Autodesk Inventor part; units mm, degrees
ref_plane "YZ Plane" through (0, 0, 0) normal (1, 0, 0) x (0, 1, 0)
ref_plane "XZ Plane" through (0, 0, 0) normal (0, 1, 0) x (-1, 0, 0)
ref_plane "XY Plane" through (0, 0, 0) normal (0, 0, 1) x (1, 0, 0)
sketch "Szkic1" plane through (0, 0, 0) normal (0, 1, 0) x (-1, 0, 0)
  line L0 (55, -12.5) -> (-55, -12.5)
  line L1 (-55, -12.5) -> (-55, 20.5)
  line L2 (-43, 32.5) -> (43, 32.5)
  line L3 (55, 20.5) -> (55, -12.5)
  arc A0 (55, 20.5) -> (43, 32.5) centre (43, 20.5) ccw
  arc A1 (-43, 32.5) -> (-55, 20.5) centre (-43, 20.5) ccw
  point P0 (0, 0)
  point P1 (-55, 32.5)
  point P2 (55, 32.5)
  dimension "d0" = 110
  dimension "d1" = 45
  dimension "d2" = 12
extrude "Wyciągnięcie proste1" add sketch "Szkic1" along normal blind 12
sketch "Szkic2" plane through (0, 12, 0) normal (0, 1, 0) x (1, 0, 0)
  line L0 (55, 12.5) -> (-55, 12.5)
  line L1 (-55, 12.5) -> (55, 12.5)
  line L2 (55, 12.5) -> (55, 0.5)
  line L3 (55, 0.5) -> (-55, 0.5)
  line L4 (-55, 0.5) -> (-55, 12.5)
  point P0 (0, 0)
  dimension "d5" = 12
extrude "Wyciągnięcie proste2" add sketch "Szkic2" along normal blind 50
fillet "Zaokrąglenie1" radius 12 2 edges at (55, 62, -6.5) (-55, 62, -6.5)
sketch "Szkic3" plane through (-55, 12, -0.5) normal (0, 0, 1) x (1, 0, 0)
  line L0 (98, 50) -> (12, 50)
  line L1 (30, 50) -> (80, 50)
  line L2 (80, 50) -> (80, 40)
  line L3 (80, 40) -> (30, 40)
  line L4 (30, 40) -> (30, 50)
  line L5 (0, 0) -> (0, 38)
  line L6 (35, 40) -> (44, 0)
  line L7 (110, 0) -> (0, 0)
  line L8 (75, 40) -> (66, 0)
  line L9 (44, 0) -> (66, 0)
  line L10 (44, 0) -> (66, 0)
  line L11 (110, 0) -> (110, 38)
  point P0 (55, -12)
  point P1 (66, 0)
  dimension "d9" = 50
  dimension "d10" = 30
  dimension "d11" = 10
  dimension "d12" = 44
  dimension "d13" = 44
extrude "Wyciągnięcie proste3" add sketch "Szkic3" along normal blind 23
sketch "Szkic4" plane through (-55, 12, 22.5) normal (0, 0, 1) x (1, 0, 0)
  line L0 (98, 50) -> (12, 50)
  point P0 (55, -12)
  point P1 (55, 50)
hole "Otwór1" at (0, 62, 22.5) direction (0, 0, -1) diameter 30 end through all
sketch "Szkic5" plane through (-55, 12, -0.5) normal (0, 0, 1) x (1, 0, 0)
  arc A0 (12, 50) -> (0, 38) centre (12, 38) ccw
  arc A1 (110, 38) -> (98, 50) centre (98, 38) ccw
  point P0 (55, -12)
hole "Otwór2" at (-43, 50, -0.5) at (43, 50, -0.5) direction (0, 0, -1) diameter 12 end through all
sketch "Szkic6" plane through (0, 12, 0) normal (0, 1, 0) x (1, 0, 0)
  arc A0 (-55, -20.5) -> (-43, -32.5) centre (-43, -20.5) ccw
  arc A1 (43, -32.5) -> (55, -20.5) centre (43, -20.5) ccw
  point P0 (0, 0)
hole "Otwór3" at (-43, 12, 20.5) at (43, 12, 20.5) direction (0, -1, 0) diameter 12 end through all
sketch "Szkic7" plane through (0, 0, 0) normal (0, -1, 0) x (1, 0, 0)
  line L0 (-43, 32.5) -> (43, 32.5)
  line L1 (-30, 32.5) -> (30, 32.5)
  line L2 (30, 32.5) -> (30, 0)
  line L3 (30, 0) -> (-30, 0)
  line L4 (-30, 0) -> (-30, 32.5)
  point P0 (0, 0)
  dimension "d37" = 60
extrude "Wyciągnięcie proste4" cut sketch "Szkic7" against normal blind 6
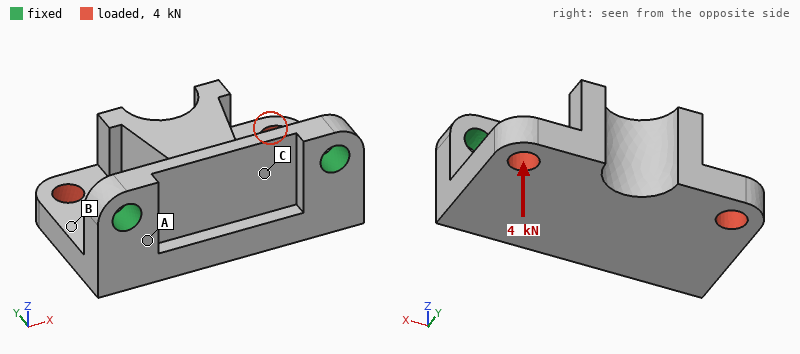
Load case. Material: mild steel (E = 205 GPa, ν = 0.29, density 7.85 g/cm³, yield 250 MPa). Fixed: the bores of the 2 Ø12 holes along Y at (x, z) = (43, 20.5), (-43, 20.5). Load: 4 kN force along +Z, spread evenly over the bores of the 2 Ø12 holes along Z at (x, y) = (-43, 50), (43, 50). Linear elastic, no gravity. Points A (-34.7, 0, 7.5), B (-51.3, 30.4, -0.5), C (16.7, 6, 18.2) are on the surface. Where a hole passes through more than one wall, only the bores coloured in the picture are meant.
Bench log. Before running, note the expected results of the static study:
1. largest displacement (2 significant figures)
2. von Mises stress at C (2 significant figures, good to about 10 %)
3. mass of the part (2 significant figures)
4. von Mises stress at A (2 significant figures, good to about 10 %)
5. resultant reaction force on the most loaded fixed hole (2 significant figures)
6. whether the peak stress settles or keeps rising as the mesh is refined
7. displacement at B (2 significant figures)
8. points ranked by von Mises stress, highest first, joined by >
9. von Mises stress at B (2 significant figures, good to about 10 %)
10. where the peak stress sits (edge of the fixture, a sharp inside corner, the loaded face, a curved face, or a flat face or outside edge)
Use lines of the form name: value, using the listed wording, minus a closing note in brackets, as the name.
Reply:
largest displacement: 0.13 mm
von Mises stress at C: 58 MPa
mass of the part: 1.1 kg
von Mises stress at A: 90 MPa
resultant reaction force on the most loaded fixed hole: 2.2 kN
whether the peak stress settles or keeps rising as the mesh is refined: keeps rising
displacement at B: 0.050 mm
points ranked by von Mises stress, highest first, joined by >: A > C > B
von Mises stress at B: 21 MPa
where the peak stress sits: edge of the fixture
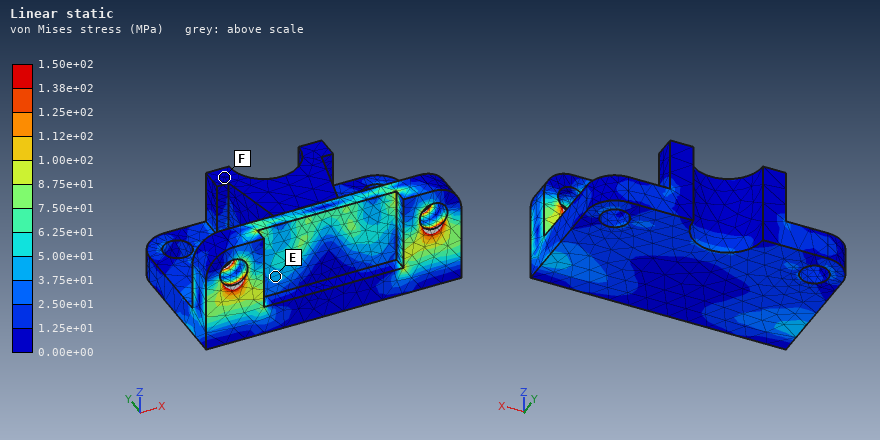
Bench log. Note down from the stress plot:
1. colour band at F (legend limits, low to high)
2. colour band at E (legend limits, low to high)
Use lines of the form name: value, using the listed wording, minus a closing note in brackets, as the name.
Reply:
colour band at F: 0.00e+00 to 1.25e+01 MPa
colour band at E: 3.75e+01 to 5.00e+01 MPa
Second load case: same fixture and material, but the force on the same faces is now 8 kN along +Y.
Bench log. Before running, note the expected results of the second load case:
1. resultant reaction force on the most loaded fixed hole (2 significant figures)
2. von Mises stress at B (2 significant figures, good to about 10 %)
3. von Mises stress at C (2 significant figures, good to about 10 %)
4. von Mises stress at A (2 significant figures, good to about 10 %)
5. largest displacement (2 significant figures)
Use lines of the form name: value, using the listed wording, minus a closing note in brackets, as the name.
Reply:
resultant reaction force on the most loaded fixed hole: 4.0 kN
von Mises stress at B: 19 MPa
von Mises stress at C: 27 MPa
von Mises stress at A: 66 MPa
largest displacement: 71 µm
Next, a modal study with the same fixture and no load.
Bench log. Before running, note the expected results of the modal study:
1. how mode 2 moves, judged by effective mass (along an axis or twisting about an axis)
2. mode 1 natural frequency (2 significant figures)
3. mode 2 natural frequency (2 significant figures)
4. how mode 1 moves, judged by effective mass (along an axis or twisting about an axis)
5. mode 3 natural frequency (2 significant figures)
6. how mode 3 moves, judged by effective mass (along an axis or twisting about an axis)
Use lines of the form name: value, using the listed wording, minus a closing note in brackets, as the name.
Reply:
how mode 2 moves, judged by effective mass: along X
mode 1 natural frequency: 1600 Hz
mode 2 natural frequency: 4100 Hz
how mode 1 moves, judged by effective mass: along Z
mode 3 natural frequency: 4400 Hz
how mode 3 moves, judged by effective mass: along Y
